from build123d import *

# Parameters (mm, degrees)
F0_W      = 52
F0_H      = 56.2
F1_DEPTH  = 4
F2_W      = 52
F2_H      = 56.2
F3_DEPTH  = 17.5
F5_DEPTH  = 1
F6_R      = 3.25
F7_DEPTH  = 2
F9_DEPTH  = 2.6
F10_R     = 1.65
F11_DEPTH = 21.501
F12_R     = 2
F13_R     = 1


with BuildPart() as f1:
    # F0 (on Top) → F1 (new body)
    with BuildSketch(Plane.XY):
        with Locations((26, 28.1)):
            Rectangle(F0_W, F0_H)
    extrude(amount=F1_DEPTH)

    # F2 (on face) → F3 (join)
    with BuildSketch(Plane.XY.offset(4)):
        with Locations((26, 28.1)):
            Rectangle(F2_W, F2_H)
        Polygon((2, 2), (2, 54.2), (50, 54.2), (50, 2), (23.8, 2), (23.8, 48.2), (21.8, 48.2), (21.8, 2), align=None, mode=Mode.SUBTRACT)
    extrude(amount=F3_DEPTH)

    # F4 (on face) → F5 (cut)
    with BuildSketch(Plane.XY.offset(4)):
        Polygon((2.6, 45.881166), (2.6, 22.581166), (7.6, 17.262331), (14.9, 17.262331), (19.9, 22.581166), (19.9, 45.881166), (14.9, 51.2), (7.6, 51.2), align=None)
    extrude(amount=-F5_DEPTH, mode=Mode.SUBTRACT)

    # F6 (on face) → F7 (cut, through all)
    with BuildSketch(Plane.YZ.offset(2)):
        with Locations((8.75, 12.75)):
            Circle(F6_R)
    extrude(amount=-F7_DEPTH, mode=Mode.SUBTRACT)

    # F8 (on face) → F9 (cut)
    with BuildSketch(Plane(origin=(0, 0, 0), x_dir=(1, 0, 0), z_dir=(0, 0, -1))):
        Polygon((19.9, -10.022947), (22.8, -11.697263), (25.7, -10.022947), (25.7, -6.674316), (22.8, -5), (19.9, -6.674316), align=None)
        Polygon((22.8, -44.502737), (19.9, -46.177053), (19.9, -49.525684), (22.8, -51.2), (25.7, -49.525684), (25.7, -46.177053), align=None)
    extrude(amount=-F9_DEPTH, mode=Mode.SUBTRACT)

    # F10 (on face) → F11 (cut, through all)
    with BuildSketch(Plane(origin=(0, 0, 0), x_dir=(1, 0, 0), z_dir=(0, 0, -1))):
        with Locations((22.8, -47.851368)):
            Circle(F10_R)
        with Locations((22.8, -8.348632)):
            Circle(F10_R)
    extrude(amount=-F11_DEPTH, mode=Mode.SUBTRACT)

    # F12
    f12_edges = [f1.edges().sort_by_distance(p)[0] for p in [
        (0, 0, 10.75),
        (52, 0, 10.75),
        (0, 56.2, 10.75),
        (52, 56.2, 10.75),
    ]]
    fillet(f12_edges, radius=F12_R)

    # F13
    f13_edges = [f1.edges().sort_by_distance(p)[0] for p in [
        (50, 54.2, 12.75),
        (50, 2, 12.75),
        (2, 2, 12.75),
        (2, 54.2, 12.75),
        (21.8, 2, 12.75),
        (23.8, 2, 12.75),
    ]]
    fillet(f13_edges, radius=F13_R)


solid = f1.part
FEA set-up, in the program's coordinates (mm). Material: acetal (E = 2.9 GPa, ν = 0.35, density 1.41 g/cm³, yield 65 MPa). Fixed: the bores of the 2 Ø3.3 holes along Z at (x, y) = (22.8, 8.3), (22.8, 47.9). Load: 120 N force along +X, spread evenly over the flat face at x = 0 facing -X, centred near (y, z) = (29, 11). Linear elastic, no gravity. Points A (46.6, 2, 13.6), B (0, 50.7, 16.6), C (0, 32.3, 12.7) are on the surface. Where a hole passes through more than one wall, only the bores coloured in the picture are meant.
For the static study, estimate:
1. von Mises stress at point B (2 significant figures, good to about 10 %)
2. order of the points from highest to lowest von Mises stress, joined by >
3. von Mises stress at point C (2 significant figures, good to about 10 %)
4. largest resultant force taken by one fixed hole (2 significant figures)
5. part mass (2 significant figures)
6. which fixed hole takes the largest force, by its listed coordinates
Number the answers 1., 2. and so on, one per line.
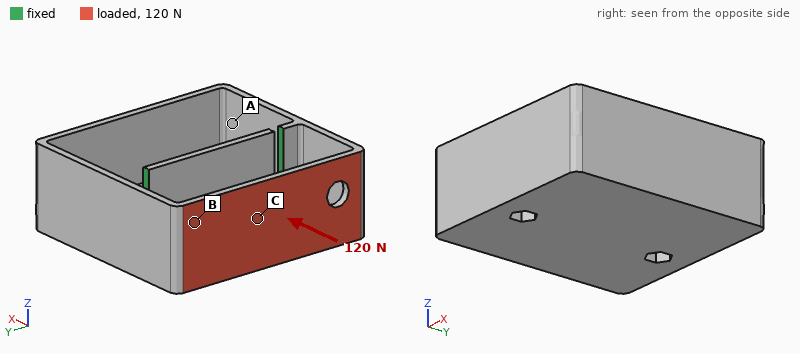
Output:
1. 7.4 MPa
2. B > C > A
3. 3.6 MPa
4. 68 N
5. 28 g
6. (22.8, 47.9)
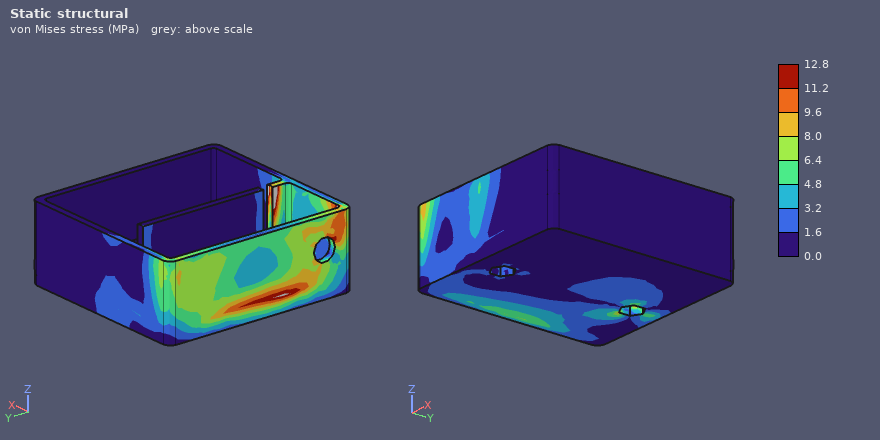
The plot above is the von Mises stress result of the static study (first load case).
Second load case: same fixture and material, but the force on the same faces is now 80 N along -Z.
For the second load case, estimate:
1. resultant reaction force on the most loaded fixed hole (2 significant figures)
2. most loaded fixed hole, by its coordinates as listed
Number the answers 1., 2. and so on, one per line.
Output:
1. 46 N
2. (22.8, 47.9)
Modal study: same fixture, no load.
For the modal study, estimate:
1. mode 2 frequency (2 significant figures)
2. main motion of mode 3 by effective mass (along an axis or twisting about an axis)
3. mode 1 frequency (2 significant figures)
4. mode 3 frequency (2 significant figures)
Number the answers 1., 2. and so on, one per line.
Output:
1. 1200 Hz
2. along Z
3. 490 Hz
4. 1600 Hz
